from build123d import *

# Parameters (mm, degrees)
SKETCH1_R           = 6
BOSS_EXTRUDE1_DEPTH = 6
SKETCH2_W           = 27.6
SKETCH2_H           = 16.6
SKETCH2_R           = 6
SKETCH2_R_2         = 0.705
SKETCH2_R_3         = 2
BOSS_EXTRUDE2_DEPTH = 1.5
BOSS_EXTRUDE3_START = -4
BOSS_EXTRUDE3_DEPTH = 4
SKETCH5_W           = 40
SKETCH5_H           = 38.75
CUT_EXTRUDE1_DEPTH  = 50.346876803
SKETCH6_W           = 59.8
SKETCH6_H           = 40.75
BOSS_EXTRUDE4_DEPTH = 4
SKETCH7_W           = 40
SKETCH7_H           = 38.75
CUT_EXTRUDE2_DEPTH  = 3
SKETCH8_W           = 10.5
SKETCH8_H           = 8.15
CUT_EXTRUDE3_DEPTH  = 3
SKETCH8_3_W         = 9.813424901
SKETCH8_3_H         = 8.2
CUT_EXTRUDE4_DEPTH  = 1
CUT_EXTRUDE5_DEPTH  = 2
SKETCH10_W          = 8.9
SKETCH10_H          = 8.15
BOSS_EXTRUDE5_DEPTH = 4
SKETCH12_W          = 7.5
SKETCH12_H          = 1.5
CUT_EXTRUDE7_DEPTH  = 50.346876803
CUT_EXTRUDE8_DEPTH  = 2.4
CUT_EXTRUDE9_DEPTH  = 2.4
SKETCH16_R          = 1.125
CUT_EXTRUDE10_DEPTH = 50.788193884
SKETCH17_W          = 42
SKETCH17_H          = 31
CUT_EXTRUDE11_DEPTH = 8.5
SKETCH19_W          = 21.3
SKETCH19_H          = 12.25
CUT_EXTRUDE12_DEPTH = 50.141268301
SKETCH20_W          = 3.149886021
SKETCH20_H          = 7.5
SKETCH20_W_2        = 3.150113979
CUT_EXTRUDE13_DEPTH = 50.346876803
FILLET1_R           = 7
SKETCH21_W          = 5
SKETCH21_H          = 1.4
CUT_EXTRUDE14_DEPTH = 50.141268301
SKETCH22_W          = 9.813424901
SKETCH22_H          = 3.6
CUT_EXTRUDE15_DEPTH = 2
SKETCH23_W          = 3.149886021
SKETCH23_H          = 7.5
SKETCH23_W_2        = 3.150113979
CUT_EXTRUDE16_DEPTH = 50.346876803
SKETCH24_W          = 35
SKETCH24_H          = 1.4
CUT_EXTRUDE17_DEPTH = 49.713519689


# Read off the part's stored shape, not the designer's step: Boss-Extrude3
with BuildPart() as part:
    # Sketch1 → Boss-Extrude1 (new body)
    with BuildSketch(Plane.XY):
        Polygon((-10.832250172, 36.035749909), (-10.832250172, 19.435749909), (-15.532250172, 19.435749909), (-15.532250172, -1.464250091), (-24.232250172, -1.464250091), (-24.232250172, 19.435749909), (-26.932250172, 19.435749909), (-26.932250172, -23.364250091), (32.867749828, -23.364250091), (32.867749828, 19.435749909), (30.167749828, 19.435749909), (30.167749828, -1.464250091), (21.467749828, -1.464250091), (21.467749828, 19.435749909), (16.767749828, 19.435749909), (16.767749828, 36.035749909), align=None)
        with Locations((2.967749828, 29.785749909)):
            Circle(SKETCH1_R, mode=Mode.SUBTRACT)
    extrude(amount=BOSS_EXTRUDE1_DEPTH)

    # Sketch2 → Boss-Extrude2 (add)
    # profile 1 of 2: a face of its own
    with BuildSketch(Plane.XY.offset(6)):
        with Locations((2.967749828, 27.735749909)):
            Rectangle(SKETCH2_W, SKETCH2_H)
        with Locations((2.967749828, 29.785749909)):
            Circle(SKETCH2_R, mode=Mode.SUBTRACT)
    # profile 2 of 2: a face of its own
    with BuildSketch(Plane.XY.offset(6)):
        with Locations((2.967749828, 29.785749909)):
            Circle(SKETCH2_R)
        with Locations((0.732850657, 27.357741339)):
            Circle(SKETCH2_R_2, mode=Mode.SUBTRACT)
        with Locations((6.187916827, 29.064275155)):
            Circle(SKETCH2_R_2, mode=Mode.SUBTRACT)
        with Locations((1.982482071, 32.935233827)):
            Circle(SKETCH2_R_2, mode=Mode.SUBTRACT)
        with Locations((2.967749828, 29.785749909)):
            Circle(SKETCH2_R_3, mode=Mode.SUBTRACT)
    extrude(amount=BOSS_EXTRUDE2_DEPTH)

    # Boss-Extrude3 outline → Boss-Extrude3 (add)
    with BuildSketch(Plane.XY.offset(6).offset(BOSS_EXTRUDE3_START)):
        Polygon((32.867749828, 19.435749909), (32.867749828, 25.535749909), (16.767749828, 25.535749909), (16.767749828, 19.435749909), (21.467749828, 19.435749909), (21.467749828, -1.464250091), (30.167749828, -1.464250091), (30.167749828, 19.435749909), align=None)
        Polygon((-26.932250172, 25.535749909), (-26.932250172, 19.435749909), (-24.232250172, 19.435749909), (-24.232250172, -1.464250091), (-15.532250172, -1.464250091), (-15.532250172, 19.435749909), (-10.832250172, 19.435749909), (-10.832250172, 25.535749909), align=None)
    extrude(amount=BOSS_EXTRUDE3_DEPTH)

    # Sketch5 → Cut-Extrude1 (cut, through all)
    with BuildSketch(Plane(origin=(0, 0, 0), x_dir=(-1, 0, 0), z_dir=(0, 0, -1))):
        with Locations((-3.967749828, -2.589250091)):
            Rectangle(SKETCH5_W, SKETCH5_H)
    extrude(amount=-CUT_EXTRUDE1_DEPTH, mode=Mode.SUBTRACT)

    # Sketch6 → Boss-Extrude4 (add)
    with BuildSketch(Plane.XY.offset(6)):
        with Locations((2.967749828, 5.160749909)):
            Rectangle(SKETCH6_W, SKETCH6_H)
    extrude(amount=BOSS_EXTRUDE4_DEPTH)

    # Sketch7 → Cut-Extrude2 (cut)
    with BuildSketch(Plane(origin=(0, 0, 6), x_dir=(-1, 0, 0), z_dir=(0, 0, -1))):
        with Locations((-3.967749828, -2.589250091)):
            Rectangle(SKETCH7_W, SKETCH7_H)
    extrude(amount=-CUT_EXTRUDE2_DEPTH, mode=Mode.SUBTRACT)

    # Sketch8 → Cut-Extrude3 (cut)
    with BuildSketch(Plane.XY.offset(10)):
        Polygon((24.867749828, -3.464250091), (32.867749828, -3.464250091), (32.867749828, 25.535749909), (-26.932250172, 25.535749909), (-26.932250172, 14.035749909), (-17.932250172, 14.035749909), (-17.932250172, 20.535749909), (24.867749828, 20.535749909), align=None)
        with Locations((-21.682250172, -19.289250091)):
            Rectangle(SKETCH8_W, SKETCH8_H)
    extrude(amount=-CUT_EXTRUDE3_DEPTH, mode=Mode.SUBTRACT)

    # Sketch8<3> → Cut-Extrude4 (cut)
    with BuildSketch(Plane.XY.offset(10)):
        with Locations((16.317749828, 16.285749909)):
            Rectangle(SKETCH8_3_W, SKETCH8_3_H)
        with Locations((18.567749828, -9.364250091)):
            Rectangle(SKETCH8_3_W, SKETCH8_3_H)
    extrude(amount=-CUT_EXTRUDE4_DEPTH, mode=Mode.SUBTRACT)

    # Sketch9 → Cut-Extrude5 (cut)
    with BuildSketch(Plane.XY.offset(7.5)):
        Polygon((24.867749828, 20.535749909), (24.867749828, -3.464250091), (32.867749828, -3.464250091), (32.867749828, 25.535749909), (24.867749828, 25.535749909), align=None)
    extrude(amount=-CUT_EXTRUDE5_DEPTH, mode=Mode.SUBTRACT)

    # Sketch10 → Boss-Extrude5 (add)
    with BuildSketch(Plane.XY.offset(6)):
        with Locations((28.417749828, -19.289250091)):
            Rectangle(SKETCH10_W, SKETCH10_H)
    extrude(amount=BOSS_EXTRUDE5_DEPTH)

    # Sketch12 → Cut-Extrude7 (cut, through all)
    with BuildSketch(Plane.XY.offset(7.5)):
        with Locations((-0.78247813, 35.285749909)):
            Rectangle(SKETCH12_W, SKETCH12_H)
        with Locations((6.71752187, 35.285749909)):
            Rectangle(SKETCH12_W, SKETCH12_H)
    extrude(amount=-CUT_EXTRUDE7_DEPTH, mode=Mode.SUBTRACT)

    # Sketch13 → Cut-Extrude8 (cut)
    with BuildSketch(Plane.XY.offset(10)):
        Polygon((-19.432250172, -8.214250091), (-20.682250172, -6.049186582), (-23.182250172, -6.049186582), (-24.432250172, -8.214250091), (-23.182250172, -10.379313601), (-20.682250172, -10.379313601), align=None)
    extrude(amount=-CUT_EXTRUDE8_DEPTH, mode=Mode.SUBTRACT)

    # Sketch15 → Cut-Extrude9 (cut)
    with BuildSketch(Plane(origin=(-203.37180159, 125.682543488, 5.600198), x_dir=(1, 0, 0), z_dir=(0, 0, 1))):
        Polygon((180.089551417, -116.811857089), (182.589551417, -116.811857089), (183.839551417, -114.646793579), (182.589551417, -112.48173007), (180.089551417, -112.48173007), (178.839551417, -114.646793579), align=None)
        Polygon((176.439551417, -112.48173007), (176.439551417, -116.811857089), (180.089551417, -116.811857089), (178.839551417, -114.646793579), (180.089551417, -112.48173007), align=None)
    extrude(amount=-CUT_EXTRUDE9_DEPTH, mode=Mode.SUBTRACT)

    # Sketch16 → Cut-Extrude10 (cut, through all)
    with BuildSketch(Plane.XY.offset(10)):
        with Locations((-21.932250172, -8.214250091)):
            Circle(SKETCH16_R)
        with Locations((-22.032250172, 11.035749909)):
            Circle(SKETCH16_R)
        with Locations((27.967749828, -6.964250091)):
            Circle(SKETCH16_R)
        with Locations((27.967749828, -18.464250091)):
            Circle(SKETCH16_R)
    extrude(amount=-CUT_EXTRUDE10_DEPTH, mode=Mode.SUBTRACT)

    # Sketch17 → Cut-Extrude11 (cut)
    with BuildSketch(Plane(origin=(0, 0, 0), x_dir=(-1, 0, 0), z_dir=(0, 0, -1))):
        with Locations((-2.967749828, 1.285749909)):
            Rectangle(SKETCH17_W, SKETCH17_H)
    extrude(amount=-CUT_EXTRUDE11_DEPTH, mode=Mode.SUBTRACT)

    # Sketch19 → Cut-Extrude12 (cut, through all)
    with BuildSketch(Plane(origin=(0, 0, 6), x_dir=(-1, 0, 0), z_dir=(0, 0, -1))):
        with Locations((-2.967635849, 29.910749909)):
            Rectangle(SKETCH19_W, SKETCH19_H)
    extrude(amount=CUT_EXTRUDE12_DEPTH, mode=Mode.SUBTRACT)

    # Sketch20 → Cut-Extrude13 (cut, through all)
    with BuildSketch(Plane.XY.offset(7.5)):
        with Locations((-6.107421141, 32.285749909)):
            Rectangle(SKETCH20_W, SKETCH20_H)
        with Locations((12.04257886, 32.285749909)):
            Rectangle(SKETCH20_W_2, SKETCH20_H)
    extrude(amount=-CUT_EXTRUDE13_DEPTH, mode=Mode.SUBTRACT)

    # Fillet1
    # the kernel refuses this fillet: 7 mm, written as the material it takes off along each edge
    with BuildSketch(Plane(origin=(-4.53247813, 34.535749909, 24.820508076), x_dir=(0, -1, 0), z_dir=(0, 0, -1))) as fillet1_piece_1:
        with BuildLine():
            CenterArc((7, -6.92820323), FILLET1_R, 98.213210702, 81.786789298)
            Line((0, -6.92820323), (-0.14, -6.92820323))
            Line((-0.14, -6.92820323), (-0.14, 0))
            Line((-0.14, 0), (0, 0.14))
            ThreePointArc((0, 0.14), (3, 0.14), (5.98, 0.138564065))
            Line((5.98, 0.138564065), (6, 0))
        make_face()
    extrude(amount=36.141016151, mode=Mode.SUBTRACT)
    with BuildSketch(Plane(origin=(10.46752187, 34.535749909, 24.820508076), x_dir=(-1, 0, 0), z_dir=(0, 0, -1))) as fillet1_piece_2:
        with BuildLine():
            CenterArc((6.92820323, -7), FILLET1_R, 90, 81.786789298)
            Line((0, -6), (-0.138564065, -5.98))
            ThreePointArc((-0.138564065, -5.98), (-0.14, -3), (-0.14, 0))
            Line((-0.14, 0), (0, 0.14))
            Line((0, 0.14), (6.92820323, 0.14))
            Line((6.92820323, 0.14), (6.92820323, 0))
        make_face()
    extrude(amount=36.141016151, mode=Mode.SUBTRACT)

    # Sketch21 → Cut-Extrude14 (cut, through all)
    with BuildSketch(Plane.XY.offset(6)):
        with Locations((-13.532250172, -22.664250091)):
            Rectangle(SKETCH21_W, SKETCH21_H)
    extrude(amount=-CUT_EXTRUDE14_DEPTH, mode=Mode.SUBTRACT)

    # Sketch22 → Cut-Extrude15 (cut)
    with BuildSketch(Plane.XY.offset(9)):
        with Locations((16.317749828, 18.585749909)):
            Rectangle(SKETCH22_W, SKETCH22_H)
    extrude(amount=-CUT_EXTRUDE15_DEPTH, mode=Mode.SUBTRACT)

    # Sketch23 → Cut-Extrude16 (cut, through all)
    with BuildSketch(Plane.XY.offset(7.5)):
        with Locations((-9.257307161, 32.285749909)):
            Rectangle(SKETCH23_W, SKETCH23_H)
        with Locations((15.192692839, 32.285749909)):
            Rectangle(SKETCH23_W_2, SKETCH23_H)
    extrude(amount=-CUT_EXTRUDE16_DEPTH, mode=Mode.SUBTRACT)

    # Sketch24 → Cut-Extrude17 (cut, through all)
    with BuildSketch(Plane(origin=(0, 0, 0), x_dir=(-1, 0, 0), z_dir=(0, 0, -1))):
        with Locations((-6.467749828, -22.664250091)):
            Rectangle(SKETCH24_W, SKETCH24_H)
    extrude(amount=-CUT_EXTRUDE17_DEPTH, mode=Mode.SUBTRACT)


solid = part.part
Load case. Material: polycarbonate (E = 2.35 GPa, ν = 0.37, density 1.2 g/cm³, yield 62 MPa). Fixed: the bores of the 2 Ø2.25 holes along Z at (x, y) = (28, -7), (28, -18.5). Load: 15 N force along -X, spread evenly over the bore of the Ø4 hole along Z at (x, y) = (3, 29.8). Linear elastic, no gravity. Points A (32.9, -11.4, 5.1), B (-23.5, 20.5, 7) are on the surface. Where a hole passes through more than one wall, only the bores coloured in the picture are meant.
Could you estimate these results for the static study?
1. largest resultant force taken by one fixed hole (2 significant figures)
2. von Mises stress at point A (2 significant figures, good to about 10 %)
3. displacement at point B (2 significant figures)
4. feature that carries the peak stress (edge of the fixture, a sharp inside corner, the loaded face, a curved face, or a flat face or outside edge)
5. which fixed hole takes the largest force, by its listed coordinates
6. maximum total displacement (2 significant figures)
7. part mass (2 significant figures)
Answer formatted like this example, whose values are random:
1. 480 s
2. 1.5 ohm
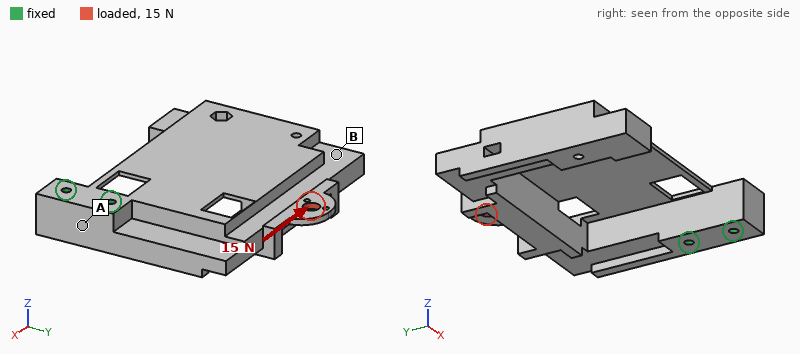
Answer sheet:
1. 49 N
2. 1.5 MPa
3. 0.76 mm
4. a flat face or outside edge
5. (28, -7)
6. 0.85 mm
7. 12 g
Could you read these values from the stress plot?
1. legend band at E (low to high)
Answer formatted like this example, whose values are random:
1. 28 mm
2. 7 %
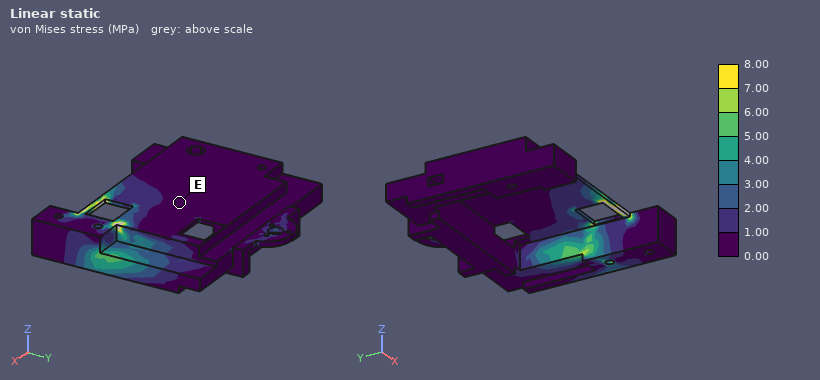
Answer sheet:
1. 0.00 to 1.00 MPa
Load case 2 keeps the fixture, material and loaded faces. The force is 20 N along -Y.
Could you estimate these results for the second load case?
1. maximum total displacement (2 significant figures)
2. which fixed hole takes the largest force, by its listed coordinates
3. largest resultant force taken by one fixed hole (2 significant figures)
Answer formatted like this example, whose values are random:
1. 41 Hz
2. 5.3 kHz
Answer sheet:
1. 0.88 mm
2. (28, -7)
3. 37 N
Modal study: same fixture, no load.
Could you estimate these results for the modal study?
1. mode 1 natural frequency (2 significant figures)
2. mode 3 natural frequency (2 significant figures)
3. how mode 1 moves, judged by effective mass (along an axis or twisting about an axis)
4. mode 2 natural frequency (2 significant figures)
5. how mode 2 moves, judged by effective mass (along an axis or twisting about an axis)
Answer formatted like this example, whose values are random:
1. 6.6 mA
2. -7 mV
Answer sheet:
1. 100 Hz
2. 430 Hz
3. along Z
4. 250 Hz
5. along Y
